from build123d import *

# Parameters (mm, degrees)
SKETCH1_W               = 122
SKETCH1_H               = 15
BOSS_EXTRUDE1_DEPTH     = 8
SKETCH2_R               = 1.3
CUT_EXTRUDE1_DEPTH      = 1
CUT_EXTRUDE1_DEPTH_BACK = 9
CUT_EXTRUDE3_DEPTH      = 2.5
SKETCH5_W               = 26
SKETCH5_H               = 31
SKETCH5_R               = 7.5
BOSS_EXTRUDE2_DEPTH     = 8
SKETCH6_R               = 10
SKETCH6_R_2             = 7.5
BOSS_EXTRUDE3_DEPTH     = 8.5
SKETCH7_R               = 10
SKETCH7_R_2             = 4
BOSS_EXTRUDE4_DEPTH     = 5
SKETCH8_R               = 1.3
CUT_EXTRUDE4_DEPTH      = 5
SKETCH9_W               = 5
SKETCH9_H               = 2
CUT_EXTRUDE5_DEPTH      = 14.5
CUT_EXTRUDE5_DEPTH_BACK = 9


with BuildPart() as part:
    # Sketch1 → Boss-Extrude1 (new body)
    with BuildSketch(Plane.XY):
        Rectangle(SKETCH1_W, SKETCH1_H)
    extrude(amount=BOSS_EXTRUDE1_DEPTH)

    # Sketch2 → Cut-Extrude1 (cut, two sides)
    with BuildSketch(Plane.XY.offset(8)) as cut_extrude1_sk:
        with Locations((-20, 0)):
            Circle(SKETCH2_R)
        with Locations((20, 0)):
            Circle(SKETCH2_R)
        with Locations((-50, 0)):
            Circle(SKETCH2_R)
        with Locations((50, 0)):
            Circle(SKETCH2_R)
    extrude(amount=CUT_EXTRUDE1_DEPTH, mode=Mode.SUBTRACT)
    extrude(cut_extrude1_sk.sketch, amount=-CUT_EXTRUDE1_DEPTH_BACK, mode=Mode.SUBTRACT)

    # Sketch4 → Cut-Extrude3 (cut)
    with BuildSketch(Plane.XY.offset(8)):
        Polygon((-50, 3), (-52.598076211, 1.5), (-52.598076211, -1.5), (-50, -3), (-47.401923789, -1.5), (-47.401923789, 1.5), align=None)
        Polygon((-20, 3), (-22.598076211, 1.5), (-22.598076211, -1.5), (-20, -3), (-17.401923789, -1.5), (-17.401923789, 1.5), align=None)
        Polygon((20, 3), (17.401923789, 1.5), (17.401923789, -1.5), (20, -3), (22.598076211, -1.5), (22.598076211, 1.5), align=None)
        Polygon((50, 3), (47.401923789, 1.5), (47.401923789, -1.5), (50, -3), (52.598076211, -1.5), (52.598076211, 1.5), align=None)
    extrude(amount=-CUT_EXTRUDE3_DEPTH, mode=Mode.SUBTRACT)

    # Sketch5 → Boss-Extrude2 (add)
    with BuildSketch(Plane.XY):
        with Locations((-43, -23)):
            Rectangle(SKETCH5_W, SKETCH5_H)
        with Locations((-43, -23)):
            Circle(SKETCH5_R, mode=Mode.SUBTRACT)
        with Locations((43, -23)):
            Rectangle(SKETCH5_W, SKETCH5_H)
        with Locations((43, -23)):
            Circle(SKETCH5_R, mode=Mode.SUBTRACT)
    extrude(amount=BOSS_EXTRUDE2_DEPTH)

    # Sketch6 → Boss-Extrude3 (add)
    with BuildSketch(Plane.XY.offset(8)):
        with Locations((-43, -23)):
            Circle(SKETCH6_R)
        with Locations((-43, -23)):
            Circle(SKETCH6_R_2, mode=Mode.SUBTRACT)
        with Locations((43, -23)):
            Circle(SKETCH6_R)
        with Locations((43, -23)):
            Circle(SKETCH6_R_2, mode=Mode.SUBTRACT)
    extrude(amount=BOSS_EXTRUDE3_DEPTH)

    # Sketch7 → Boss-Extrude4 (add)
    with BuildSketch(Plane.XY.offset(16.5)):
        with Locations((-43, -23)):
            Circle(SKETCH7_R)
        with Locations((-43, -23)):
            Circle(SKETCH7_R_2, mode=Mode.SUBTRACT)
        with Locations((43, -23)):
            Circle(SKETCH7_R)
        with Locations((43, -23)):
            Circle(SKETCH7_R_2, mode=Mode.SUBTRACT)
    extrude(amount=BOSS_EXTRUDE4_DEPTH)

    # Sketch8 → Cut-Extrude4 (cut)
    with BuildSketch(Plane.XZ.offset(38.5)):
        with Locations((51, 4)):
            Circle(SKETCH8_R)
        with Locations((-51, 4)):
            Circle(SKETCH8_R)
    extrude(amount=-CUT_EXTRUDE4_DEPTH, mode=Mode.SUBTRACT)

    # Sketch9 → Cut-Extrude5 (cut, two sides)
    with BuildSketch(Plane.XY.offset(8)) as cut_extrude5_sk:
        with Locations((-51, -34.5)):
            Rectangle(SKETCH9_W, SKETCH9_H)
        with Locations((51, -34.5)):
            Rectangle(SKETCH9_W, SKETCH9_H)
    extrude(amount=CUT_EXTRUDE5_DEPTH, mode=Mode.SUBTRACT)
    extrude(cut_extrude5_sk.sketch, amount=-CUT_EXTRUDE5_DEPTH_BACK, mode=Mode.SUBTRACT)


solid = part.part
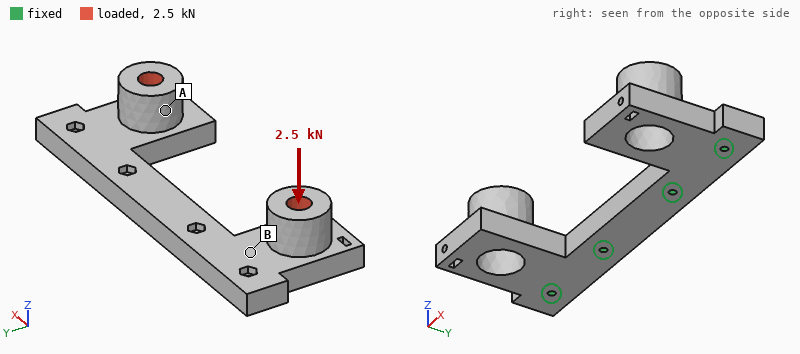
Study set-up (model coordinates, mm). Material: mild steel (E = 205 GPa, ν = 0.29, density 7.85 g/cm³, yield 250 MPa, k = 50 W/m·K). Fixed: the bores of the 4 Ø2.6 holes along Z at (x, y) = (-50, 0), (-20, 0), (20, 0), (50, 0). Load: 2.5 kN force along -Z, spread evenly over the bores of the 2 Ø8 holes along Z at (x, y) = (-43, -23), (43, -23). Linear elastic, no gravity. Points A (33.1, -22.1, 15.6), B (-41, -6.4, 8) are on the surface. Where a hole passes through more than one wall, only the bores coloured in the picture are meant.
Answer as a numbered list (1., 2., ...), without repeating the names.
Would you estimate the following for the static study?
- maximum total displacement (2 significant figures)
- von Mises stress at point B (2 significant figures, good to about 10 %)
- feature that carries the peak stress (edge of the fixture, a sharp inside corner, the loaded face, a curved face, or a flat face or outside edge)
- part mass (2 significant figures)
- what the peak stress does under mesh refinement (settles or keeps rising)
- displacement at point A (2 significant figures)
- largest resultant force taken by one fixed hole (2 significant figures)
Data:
1. 95 µm
2. 60 MPa
3. edge of the fixture
4. 230 g
5. keeps rising
6. 59 µm
7. 960 N
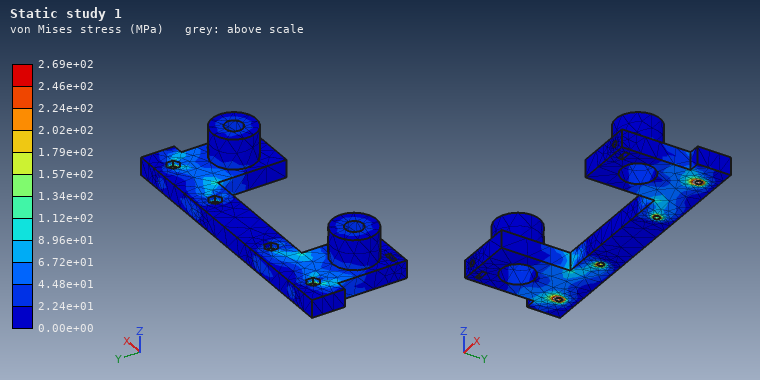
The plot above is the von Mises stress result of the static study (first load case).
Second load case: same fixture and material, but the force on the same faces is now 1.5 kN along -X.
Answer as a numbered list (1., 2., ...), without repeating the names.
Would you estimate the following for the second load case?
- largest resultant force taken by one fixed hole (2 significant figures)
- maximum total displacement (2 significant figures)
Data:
1. 920 N
2. 19 µm
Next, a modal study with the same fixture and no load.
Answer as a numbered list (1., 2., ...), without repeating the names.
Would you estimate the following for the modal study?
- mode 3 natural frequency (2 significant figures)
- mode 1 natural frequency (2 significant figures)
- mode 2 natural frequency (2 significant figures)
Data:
1. 7100 Hz
2. 2800 Hz
3. 2800 Hz
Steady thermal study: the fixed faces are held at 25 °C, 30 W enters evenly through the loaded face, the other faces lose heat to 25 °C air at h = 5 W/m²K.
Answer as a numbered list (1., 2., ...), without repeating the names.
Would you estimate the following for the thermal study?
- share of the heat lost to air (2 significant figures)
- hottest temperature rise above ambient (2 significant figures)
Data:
1. 6.1 %
2. 68 K
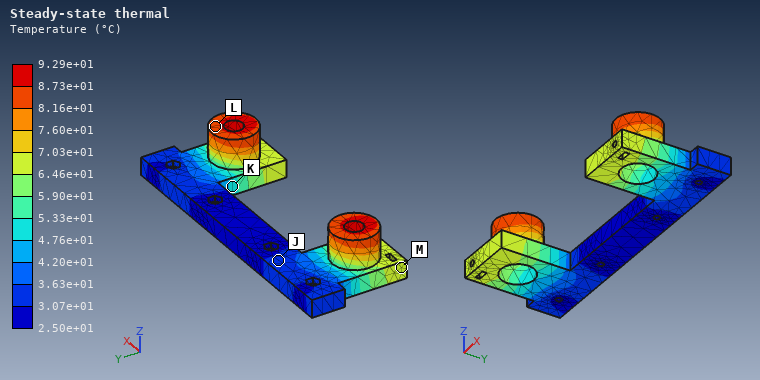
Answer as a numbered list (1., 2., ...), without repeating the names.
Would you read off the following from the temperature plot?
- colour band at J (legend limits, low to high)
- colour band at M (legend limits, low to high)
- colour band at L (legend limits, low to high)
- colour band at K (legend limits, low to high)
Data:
1. 3.07e+01 to 3.63e+01 °C
2. 6.46e+01 to 7.03e+01 °C
3. 8.16e+01 to 8.73e+01 °C
4. 4.76e+01 to 5.33e+01 °C
